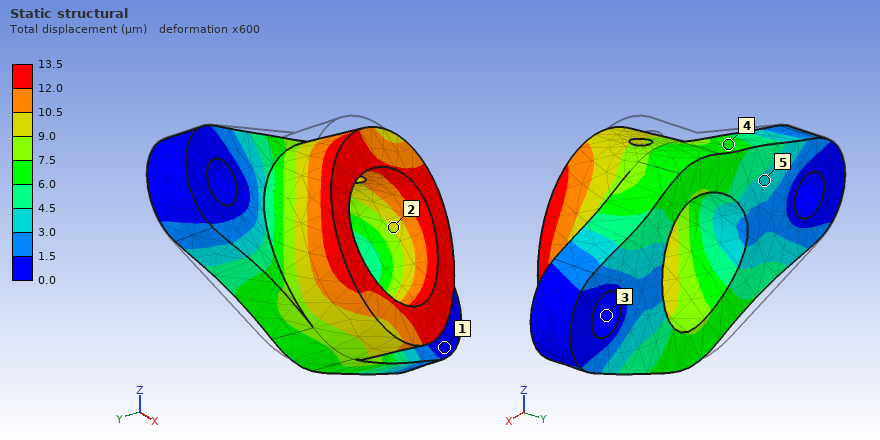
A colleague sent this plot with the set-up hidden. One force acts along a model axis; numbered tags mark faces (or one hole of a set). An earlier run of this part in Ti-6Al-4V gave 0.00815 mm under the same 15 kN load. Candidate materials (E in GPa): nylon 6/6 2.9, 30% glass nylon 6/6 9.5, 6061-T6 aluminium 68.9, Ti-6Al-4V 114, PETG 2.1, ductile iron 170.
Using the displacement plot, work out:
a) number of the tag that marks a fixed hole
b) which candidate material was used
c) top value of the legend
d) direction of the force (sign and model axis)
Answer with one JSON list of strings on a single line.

["3", "6061-T6 aluminium", "13.5 µm", "+X"]
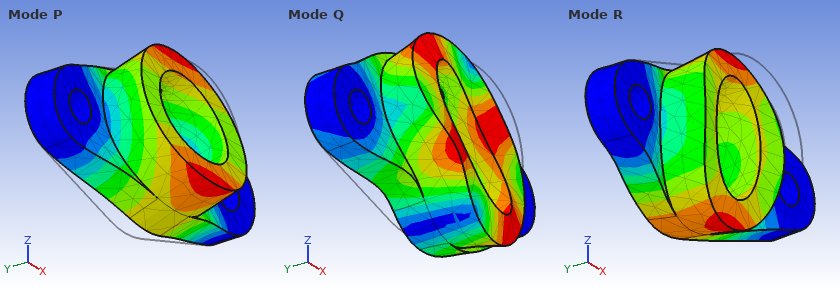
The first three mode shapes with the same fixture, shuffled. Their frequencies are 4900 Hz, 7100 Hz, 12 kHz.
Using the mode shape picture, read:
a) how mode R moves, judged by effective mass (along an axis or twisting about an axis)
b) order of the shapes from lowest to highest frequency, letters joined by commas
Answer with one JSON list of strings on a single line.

["along Y", "P, R, Q"]
